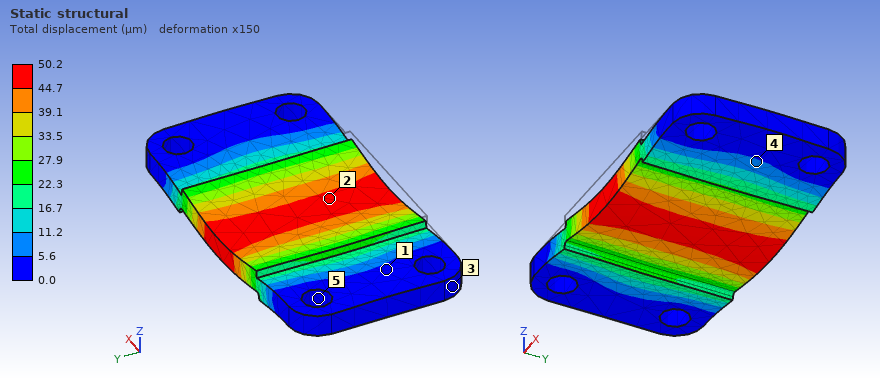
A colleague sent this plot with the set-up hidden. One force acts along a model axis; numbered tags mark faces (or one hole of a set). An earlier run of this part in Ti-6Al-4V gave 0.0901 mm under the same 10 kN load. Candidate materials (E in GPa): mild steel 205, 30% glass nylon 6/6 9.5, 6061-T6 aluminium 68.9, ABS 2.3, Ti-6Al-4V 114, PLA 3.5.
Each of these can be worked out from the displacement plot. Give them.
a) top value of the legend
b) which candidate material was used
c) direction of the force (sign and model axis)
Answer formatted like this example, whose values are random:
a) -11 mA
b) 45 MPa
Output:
a) 50.2 µm
b) mild steel
c) -Z
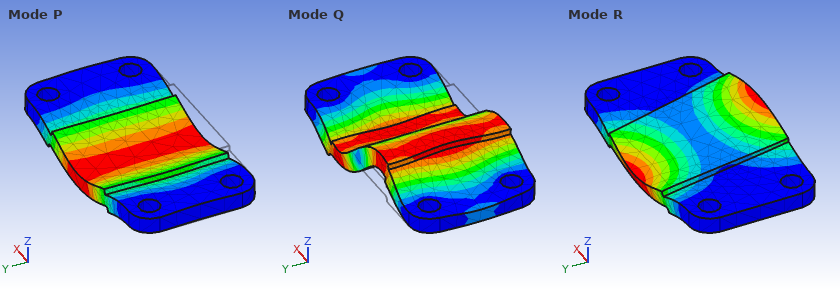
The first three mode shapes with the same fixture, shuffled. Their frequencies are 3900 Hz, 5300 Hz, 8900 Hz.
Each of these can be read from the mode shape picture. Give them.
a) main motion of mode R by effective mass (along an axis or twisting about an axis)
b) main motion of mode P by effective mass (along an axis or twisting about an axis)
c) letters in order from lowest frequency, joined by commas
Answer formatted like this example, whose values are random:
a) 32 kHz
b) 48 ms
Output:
a) twisting about X
b) along Z
c) P, R, Q
